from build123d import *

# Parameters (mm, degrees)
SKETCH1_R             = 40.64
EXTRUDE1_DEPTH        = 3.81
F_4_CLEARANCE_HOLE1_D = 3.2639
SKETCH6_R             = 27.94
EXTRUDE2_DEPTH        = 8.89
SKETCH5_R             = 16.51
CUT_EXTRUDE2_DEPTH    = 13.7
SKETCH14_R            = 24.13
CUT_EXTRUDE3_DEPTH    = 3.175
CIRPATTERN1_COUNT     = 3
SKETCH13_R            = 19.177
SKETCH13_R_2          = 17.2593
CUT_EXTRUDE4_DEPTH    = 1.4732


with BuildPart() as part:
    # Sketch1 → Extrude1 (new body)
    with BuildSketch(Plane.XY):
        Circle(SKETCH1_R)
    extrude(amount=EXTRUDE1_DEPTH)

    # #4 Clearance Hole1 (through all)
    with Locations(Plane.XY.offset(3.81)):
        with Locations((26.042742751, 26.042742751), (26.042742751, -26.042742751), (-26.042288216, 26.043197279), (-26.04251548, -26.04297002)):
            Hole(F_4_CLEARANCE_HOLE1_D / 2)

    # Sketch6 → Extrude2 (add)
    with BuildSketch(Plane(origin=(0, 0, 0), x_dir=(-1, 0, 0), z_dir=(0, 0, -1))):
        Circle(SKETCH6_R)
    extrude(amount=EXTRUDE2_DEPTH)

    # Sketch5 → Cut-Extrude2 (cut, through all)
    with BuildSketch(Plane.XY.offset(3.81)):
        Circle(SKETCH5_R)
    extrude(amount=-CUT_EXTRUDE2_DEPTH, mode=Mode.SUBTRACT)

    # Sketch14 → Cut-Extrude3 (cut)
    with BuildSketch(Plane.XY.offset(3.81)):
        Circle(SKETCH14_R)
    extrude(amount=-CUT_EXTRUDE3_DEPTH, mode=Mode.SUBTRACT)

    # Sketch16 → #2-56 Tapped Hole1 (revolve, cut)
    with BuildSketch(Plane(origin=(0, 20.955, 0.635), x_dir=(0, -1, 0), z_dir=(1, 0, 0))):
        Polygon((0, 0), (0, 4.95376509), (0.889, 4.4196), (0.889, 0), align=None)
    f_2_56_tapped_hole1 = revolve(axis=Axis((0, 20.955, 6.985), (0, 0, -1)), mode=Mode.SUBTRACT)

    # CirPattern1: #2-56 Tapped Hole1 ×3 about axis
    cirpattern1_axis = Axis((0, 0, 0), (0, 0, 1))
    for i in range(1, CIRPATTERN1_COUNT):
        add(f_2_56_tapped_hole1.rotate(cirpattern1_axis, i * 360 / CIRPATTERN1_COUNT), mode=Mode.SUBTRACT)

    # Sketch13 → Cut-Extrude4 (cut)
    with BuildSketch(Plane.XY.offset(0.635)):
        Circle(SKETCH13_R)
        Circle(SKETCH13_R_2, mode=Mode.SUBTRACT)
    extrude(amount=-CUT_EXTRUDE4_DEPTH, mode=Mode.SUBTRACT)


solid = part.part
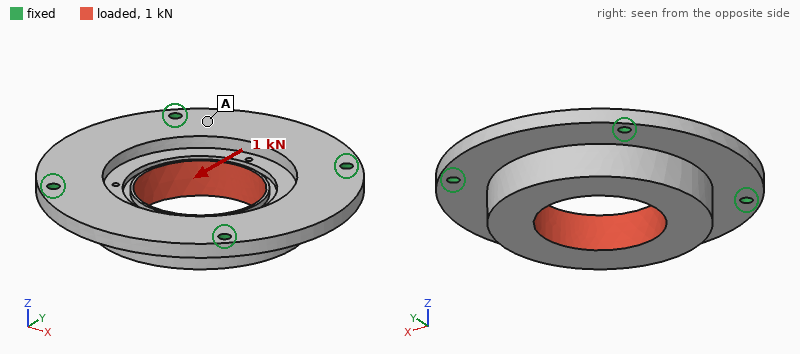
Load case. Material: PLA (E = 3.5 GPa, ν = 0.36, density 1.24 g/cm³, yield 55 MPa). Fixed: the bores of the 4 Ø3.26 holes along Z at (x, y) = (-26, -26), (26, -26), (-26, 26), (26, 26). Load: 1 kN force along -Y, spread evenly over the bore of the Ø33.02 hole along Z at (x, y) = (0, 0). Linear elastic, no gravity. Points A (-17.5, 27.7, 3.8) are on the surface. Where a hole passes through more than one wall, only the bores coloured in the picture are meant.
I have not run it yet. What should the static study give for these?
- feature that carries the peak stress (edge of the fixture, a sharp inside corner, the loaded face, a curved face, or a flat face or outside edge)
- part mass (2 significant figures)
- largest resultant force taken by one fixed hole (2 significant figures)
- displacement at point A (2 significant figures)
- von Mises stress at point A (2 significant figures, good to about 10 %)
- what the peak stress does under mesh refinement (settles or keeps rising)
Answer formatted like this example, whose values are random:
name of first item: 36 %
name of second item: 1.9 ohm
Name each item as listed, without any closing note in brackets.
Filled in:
feature that carries the peak stress: edge of the fixture
part mass: 34 g
largest resultant force taken by one fixed hole: 260 N
displacement at point A: 28 µm
von Mises stress at point A: 1.9 MPa
what the peak stress does under mesh refinement: keeps rising
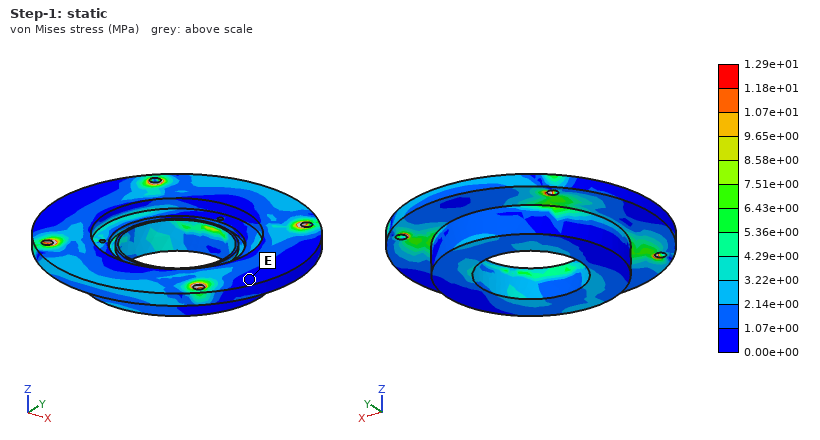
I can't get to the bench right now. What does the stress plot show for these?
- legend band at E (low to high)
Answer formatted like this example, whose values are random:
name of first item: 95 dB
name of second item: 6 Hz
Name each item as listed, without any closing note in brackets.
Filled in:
legend band at E: 0.00e+00 to 1.07e+00 MPa
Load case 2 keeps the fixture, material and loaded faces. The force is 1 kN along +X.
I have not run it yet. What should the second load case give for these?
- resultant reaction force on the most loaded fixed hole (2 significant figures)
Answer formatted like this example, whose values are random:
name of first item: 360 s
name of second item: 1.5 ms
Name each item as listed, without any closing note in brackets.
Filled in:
resultant reaction force on the most loaded fixed hole: 260 N
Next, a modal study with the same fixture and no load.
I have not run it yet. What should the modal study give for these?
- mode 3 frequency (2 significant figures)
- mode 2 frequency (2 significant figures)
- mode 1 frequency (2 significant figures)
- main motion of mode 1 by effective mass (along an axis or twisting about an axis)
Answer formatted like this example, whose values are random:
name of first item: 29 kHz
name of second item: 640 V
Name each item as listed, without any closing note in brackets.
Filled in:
mode 3 frequency: 2600 Hz
mode 2 frequency: 2600 Hz
mode 1 frequency: 2300 Hz
main motion of mode 1 by effective mass: along Z
